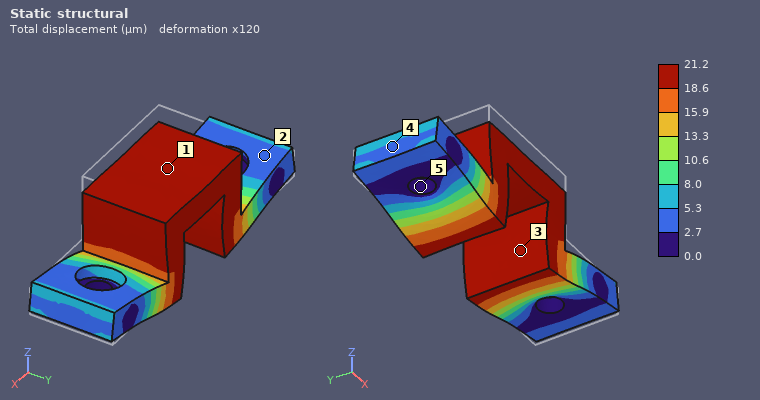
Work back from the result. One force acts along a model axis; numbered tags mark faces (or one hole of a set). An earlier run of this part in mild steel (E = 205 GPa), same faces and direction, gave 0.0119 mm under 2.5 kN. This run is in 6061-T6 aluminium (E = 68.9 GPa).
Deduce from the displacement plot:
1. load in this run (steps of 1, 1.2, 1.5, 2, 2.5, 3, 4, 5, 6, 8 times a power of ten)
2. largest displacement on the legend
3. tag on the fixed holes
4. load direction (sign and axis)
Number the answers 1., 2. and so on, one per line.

1. 1.5 kN
2. 21.2 µm
3. 5
4. -Z
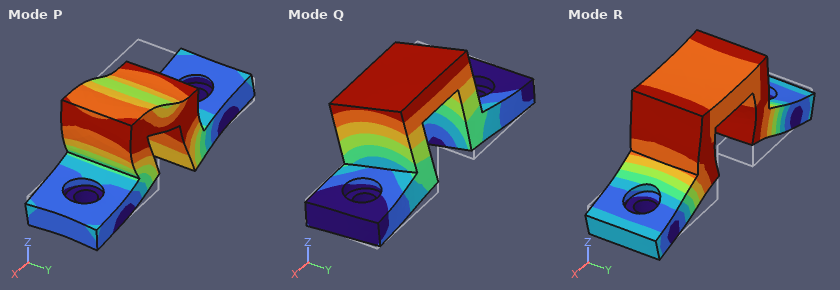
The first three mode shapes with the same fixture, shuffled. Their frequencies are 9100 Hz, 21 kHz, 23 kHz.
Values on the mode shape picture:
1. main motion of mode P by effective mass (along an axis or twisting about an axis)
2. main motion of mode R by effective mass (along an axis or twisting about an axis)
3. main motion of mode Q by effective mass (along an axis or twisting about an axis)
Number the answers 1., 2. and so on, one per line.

1. along X
2. along Z
3. along Y
